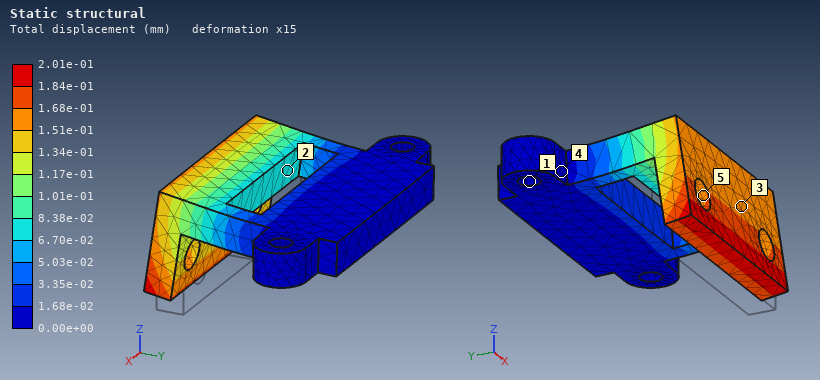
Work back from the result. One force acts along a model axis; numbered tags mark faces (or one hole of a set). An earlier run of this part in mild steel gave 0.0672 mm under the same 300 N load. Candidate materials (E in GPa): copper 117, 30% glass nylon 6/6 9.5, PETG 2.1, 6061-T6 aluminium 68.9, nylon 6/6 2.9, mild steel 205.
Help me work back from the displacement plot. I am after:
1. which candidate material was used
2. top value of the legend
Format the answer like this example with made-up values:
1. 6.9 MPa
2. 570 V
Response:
1. 6061-T6 aluminium
2. 2.01e-01 mm
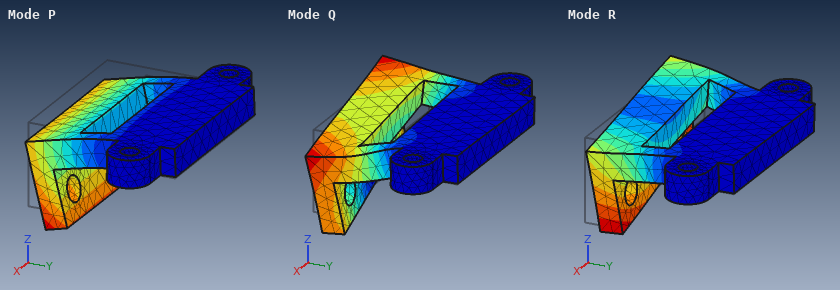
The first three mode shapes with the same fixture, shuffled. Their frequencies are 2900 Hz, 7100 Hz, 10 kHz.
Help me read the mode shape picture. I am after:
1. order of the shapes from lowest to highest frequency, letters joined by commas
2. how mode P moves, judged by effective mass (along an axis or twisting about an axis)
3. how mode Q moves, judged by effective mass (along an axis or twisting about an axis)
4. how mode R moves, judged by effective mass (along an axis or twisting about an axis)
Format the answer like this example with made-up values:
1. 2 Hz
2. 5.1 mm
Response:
1. P, R, Q
2. along Z
3. along X
4. along X
